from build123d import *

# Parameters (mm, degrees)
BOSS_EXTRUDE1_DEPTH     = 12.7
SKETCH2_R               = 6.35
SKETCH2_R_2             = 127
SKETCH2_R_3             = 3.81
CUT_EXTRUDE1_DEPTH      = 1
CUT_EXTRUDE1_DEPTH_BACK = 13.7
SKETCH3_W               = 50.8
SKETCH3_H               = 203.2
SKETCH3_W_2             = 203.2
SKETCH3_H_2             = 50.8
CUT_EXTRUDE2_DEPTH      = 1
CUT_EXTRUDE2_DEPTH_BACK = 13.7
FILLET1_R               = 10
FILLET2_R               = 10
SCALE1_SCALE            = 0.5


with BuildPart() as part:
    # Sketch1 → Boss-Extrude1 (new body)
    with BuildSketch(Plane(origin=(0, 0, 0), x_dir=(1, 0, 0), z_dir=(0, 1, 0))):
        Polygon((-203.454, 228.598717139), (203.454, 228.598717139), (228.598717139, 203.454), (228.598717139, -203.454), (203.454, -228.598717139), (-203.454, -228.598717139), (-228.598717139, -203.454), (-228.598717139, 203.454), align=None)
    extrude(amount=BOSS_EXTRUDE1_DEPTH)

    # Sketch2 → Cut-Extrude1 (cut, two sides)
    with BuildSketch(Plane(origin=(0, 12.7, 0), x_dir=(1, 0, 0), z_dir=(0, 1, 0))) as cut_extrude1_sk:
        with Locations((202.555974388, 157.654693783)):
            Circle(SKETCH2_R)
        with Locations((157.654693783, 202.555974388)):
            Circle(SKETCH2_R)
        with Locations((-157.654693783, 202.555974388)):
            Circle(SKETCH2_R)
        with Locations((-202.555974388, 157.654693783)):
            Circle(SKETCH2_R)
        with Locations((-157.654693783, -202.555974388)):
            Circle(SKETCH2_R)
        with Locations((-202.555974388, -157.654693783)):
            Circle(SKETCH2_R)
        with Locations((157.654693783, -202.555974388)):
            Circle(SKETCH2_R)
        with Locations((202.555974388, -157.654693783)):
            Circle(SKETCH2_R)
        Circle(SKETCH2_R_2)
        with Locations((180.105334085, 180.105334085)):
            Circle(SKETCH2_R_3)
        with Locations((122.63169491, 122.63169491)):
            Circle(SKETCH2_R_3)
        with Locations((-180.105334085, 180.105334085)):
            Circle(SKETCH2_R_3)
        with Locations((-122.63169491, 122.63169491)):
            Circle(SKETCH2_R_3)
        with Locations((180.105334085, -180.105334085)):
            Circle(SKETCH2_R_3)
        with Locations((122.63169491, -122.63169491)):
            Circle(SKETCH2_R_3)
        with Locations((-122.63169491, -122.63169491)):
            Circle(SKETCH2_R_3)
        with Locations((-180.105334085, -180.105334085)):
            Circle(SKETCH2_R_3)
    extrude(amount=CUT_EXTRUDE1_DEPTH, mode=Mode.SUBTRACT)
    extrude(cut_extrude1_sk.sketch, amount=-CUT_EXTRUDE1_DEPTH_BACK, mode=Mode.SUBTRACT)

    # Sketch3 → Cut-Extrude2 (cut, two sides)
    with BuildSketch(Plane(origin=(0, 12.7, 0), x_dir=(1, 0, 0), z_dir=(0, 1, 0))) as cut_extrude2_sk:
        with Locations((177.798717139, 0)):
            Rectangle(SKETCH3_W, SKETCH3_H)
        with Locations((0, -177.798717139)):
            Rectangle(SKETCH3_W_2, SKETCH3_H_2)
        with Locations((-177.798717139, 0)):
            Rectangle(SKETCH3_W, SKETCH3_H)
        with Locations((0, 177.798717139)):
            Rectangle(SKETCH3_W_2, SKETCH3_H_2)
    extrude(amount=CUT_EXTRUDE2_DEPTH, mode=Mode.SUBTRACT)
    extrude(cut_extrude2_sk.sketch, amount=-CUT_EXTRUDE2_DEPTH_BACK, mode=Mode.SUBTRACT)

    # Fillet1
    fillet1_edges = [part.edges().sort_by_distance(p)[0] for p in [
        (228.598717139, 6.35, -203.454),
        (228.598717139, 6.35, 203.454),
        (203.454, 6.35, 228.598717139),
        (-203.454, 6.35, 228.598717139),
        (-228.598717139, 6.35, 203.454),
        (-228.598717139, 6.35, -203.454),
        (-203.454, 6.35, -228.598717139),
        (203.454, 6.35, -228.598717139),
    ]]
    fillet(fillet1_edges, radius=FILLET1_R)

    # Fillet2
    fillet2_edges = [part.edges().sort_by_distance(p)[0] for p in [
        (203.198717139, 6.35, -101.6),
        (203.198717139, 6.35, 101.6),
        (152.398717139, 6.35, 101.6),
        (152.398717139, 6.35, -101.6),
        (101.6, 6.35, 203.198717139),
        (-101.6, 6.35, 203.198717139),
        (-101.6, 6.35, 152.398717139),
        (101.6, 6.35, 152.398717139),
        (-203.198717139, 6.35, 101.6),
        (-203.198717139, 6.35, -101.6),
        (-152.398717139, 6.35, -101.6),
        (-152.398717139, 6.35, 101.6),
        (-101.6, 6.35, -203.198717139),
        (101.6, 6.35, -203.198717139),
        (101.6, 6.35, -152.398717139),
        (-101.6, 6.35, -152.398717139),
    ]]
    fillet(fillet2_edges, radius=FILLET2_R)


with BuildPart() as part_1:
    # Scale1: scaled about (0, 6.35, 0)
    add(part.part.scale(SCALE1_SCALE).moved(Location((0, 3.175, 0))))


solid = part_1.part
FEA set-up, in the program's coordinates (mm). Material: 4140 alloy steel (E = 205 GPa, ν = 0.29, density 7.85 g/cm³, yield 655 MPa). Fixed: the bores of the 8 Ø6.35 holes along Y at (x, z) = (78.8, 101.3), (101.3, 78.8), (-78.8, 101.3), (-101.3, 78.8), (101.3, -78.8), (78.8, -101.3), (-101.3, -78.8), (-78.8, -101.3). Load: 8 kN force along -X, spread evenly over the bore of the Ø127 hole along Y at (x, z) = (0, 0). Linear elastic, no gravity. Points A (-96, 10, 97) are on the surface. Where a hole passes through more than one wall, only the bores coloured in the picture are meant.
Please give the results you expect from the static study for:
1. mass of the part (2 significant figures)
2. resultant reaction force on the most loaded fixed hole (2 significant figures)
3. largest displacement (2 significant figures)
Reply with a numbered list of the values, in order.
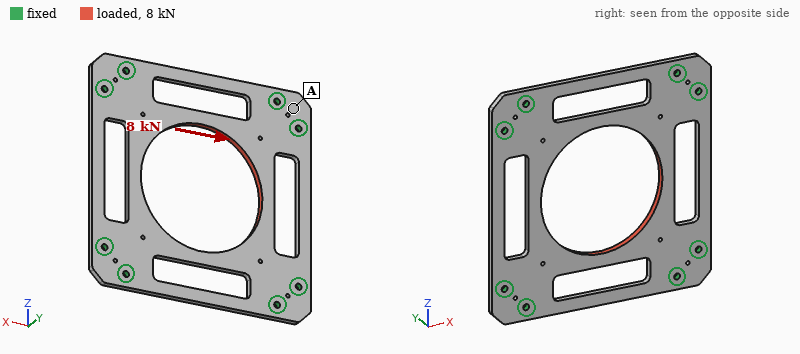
1. 1.4 kg
2. 2.5 kN
3. 19 µm
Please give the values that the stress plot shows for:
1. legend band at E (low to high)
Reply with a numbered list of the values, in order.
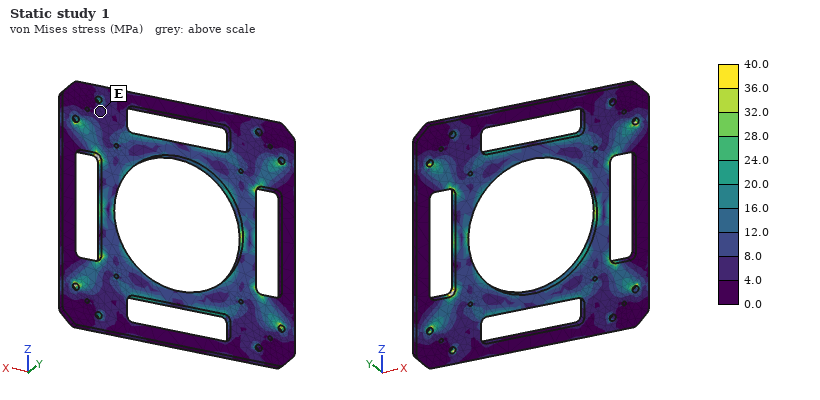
1. 4.0 to 8.0 MPa
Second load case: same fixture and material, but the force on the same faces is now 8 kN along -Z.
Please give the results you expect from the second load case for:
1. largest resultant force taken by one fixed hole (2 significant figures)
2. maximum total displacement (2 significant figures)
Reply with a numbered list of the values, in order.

1. 2.5 kN
2. 19 µm
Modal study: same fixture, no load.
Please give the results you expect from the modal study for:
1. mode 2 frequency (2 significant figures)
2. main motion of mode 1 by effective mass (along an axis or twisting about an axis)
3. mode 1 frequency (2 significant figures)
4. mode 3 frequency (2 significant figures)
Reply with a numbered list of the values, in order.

1. 1400 Hz
2. along Y
3. 1100 Hz
4. 1400 Hz
